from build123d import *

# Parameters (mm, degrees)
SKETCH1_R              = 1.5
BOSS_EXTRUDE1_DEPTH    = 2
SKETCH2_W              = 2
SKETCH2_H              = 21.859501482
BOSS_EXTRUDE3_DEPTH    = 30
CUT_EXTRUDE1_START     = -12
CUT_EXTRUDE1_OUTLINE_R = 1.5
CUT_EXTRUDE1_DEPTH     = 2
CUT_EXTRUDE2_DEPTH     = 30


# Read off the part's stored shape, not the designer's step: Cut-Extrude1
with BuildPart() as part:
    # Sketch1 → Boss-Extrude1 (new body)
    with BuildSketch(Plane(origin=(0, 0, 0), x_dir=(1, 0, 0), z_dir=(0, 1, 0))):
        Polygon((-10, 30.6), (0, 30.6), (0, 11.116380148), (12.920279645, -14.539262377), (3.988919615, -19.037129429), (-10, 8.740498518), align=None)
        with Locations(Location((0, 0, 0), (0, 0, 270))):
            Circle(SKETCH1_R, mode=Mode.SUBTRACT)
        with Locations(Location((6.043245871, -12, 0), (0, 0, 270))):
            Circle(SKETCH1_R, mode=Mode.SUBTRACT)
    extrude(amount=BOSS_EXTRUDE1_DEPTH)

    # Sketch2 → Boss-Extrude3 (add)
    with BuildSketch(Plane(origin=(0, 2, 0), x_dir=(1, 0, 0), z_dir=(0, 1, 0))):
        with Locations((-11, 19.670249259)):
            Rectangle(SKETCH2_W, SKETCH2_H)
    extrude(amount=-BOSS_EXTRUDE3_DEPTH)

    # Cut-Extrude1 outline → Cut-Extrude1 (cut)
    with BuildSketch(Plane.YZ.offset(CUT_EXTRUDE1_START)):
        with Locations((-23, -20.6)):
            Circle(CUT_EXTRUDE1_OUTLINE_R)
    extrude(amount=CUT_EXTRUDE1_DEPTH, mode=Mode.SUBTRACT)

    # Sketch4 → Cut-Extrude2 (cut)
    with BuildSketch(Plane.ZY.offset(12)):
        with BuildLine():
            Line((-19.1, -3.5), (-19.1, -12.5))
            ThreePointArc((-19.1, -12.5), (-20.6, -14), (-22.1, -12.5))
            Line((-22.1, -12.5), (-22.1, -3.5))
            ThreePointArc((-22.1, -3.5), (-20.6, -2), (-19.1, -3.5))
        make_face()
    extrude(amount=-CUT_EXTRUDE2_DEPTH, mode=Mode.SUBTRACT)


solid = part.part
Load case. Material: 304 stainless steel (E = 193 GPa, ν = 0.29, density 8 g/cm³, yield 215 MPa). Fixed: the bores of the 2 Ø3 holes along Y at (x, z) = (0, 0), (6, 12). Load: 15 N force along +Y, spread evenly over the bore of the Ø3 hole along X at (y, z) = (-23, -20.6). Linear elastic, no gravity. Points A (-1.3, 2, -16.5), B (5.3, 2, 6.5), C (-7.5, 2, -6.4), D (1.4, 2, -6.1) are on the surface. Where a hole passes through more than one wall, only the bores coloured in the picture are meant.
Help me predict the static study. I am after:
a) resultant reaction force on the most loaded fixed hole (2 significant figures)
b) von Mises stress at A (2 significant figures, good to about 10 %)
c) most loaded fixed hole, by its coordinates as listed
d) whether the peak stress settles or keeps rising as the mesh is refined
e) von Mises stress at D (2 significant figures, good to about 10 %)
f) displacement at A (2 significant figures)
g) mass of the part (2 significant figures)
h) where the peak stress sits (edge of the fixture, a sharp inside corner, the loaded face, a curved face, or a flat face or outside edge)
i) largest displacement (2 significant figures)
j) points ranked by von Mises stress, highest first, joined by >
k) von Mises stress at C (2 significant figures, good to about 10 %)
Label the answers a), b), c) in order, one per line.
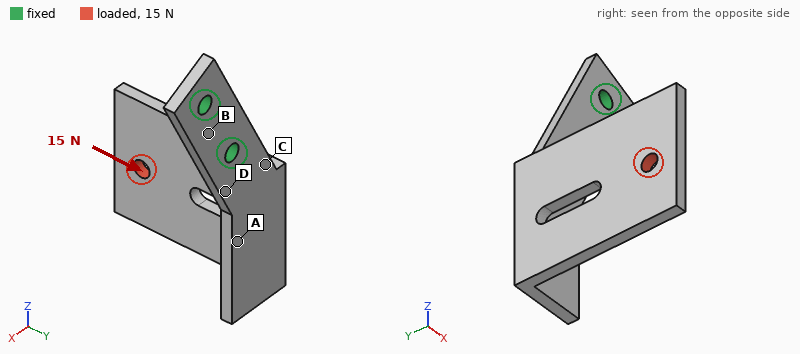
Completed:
a) 17 N
b) 9.4 MPa
c) (0, 0)
d) keeps rising
e) 40 MPa
f) 0.021 mm
g) 18 g
h) edge of the fixture
i) 0.10 mm
j) D > C > A > B
k) 33 MPa
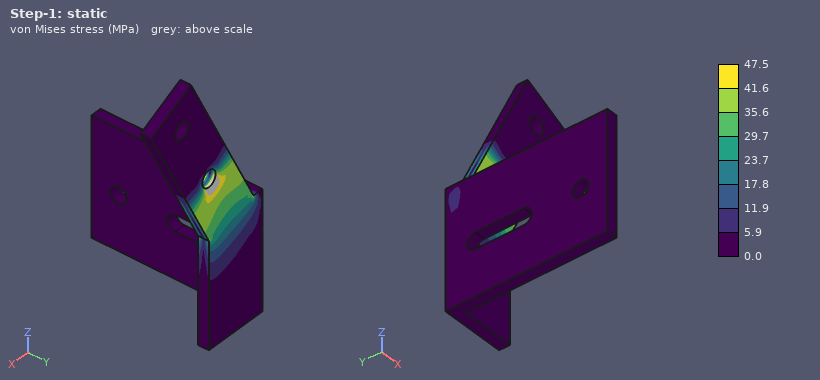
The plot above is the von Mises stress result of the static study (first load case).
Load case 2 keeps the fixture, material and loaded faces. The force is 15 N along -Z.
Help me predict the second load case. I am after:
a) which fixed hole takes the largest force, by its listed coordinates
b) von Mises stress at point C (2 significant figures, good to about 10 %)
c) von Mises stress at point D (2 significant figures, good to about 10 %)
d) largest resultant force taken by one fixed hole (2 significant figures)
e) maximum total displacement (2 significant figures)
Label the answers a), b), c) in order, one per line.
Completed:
a) (0, 0)
b) 53 MPa
c) 53 MPa
d) 18 N
e) 0.14 mm
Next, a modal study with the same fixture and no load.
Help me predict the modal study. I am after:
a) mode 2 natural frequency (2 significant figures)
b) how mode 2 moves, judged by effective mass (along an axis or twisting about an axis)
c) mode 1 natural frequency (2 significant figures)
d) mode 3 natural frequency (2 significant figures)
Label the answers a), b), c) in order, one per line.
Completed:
a) 910 Hz
b) along X
c) 610 Hz
d) 3200 Hz
